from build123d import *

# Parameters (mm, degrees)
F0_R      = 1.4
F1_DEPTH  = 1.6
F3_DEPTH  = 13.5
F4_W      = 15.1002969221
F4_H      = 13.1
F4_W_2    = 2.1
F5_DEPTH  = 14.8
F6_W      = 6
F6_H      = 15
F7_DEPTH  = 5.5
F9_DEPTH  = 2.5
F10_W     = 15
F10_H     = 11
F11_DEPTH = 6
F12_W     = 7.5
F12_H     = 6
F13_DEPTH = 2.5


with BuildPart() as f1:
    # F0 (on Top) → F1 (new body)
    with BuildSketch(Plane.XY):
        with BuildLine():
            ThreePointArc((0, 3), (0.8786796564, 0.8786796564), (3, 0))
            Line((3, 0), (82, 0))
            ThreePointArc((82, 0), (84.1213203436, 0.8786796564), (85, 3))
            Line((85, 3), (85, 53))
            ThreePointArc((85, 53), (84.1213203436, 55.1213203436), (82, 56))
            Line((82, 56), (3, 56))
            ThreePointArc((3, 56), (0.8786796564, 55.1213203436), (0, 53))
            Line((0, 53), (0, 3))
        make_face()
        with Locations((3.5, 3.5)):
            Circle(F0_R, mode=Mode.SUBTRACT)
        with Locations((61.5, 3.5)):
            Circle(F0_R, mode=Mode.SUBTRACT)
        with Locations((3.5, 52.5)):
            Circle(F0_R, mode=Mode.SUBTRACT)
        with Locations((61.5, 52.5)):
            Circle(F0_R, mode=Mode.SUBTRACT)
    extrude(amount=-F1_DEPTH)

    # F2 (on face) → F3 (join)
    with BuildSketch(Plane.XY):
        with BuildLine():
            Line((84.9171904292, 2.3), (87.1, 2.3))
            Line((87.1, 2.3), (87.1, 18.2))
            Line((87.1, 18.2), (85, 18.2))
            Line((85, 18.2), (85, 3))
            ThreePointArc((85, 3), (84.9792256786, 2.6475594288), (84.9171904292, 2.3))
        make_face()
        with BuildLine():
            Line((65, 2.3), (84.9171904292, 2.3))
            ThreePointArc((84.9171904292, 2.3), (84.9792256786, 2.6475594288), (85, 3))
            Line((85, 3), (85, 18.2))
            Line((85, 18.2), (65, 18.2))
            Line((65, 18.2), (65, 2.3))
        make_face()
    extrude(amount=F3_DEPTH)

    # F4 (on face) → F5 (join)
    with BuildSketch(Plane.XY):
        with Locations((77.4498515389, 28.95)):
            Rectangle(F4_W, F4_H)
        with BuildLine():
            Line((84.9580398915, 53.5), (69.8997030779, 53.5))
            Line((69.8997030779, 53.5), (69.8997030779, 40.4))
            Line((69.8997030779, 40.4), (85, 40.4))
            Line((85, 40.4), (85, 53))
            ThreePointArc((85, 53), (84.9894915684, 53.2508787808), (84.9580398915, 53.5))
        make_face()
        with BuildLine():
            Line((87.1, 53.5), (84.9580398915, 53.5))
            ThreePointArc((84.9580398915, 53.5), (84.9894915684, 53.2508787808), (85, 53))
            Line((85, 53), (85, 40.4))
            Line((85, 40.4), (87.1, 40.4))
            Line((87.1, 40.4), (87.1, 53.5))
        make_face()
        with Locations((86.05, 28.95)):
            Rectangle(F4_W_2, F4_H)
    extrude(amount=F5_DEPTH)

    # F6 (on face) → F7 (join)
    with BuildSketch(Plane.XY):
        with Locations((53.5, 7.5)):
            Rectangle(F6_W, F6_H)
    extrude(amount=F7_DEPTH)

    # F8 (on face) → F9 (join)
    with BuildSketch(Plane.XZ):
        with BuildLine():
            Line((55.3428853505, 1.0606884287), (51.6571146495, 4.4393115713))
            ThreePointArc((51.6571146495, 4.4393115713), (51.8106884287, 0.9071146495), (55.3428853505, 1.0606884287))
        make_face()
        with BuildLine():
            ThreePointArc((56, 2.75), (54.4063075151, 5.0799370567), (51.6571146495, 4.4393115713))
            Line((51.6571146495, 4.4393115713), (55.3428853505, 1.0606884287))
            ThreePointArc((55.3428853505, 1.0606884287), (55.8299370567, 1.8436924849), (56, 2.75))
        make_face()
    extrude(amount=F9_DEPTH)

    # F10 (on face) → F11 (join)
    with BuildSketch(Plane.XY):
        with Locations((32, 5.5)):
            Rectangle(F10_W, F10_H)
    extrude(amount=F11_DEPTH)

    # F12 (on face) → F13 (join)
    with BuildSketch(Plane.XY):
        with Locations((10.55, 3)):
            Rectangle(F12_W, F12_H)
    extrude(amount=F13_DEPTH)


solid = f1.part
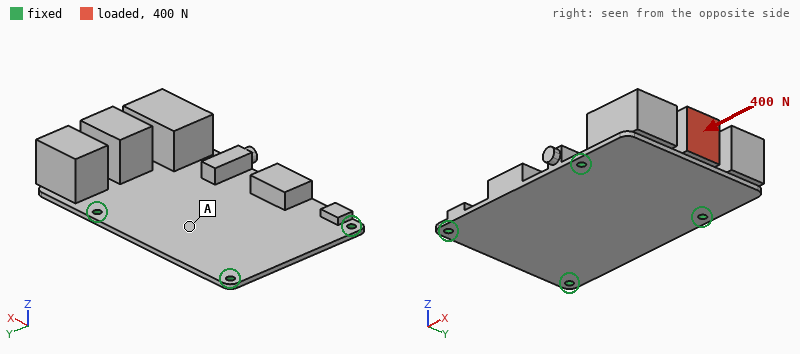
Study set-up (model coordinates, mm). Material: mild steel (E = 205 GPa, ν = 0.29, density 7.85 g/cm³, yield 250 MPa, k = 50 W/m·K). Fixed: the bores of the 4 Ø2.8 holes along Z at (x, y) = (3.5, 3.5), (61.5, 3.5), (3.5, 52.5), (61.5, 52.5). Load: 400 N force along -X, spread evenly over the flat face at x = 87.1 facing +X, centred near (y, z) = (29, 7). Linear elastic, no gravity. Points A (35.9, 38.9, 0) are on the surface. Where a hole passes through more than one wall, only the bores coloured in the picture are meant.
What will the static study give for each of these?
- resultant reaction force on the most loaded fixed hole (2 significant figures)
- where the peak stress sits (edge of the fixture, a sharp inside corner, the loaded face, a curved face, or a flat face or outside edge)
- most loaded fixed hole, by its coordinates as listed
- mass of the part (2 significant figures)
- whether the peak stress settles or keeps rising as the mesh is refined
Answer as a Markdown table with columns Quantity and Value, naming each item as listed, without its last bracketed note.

| Quantity | Value |
|---|---|
| resultant reaction force on the most loaded fixed hole | 170 N |
| where the peak stress sits | edge of the fixture |
| most loaded fixed hole, by its coordinates as listed | (61.5, 52.5) |
| mass of the part | 160 g |
| whether the peak stress settles or keeps rising as the mesh is refined | keeps rising |
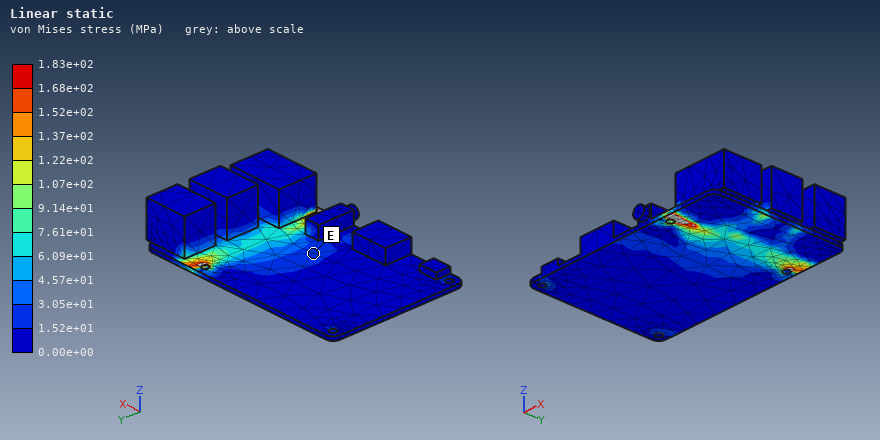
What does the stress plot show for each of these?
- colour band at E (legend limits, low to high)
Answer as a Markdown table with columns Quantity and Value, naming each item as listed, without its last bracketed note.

| Quantity | Value |
|---|---|
| colour band at E | 1.52e+01 to 3.05e+01 MPa |
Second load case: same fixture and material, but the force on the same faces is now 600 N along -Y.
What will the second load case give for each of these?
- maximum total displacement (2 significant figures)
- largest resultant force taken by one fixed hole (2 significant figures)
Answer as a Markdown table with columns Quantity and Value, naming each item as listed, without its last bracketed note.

| Quantity | Value |
|---|---|
| maximum total displacement | 67 µm |
| largest resultant force taken by one fixed hole | 450 N |
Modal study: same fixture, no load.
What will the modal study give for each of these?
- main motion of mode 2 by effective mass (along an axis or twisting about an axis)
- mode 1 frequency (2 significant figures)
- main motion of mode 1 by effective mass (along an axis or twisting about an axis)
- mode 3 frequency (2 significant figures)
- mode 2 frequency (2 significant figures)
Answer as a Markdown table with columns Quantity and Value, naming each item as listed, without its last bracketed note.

| Quantity | Value |
|---|---|
| main motion of mode 2 by effective mass | along Z |
| mode 1 frequency | 600 Hz |
| main motion of mode 1 by effective mass | along Z |
| mode 3 frequency | 2100 Hz |
| mode 2 frequency | 1800 Hz |
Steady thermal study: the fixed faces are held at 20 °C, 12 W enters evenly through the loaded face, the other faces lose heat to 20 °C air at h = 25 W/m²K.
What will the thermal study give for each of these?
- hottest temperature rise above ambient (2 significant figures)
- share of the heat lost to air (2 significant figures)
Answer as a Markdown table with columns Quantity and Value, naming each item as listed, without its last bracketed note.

| Quantity | Value |
|---|---|
| hottest temperature rise above ambient | 62 K |
| share of the heat lost to air | 44 % |
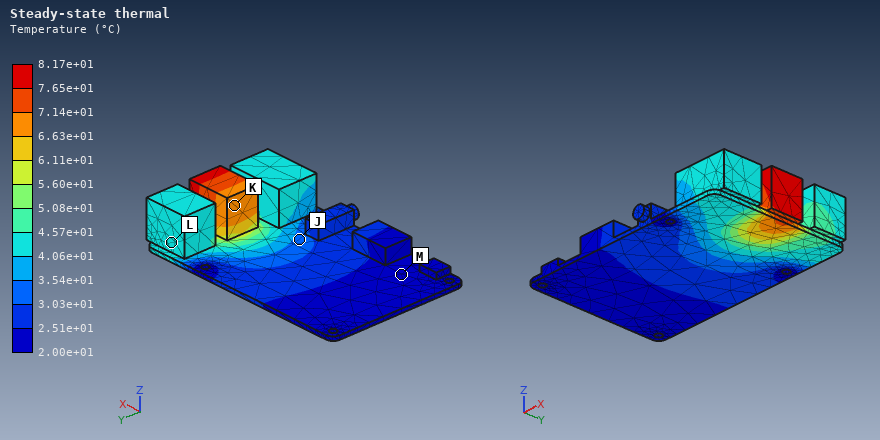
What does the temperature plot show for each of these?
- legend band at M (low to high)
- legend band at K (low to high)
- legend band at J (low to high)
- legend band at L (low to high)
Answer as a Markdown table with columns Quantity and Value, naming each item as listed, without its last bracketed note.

| Quantity | Value |
|---|---|
| legend band at M | 2.00e+01 to 2.51e+01 °C |
| legend band at K | 6.63e+01 to 7.14e+01 °C |
| legend band at J | 3.03e+01 to 3.54e+01 °C |
| legend band at L | 4.06e+01 to 4.57e+01 °C |
